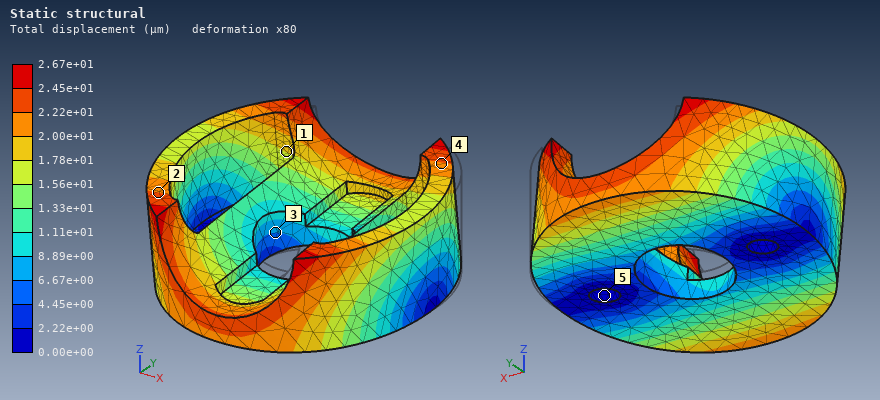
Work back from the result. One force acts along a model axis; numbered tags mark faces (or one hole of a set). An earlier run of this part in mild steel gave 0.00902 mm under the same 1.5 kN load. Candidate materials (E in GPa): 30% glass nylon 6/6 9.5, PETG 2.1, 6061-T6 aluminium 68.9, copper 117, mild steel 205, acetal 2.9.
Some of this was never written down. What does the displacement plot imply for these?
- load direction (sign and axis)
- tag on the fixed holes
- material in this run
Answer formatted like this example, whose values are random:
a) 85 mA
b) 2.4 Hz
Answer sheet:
a) -Y
b) 5
c) 6061-T6 aluminium
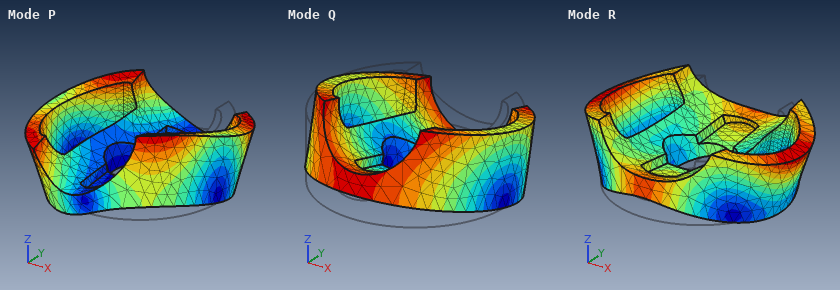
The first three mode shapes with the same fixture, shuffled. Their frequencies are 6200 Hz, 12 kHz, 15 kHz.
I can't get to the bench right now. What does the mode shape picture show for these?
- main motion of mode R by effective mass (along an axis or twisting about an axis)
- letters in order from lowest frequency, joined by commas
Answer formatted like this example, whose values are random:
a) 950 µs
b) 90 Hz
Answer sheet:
a) along Z
b) Q, R, P
